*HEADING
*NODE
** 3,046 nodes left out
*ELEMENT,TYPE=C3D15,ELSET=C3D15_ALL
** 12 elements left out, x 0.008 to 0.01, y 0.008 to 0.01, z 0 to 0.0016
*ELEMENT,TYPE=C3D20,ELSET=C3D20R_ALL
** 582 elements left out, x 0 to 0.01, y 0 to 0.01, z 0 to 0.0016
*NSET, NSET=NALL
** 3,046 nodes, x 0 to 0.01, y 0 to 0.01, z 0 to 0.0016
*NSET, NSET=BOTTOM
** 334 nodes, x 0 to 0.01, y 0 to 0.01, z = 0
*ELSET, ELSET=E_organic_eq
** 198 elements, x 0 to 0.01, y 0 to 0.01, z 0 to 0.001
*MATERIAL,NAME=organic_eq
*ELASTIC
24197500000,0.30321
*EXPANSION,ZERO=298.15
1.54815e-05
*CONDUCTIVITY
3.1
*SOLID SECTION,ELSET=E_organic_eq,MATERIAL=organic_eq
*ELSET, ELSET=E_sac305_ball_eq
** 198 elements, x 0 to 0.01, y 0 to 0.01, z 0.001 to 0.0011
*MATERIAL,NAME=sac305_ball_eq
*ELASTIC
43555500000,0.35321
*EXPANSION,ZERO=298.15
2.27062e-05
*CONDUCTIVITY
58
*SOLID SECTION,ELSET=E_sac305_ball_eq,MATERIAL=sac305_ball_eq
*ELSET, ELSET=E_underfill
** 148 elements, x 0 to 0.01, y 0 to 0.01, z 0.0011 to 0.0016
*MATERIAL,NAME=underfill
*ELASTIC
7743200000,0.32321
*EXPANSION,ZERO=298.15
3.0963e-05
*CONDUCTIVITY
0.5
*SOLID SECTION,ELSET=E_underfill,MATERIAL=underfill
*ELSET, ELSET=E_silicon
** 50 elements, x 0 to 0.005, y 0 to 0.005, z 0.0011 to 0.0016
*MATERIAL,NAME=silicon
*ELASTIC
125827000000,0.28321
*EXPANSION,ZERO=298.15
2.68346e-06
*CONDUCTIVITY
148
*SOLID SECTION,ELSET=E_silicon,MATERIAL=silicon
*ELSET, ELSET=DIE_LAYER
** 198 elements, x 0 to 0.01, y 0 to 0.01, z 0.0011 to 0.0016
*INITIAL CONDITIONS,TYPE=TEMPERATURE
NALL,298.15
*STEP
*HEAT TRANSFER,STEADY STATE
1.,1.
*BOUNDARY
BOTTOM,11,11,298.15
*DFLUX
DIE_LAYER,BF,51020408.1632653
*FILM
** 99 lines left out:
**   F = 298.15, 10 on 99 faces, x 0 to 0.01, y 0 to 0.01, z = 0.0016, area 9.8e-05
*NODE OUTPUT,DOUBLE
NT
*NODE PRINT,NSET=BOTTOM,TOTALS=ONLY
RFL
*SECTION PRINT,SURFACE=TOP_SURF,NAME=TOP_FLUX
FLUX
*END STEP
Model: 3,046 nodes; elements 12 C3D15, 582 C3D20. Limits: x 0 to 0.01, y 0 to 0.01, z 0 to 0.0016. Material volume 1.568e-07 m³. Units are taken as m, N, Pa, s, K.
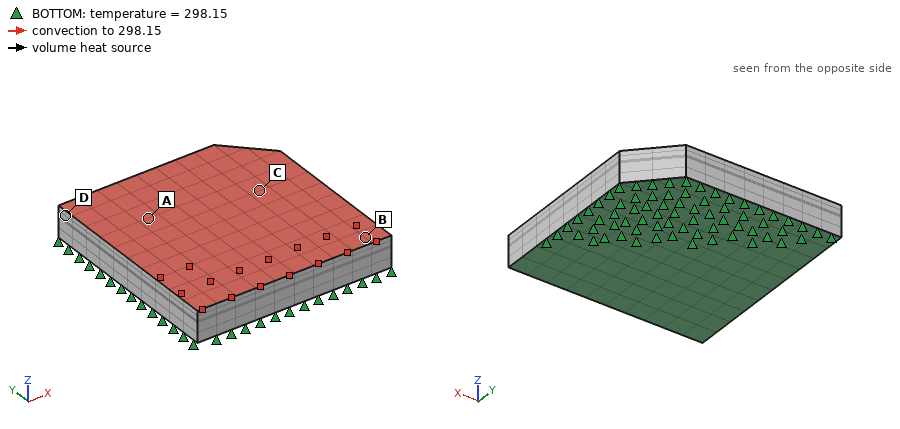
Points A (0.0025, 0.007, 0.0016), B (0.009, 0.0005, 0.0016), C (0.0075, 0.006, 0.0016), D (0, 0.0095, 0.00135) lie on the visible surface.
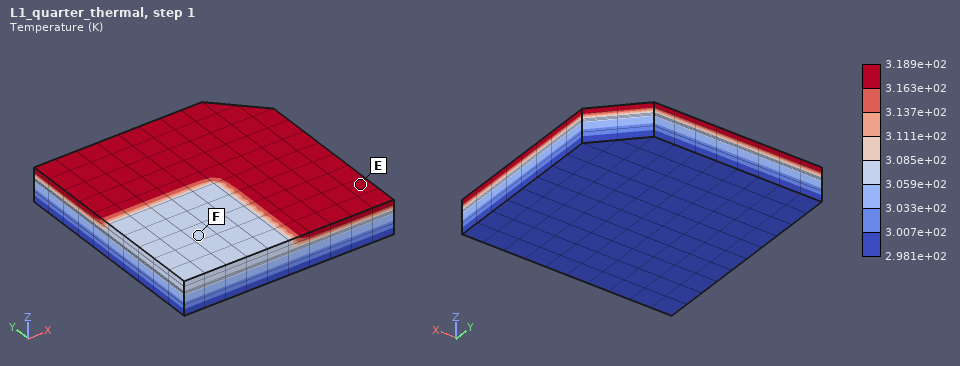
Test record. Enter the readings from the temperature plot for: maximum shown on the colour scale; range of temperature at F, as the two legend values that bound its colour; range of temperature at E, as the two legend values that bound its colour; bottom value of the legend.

3.189e+02 K
3.059e+02 to 3.085e+02 K
3.163e+02 to 3.189e+02 K
2.981e+02 K
